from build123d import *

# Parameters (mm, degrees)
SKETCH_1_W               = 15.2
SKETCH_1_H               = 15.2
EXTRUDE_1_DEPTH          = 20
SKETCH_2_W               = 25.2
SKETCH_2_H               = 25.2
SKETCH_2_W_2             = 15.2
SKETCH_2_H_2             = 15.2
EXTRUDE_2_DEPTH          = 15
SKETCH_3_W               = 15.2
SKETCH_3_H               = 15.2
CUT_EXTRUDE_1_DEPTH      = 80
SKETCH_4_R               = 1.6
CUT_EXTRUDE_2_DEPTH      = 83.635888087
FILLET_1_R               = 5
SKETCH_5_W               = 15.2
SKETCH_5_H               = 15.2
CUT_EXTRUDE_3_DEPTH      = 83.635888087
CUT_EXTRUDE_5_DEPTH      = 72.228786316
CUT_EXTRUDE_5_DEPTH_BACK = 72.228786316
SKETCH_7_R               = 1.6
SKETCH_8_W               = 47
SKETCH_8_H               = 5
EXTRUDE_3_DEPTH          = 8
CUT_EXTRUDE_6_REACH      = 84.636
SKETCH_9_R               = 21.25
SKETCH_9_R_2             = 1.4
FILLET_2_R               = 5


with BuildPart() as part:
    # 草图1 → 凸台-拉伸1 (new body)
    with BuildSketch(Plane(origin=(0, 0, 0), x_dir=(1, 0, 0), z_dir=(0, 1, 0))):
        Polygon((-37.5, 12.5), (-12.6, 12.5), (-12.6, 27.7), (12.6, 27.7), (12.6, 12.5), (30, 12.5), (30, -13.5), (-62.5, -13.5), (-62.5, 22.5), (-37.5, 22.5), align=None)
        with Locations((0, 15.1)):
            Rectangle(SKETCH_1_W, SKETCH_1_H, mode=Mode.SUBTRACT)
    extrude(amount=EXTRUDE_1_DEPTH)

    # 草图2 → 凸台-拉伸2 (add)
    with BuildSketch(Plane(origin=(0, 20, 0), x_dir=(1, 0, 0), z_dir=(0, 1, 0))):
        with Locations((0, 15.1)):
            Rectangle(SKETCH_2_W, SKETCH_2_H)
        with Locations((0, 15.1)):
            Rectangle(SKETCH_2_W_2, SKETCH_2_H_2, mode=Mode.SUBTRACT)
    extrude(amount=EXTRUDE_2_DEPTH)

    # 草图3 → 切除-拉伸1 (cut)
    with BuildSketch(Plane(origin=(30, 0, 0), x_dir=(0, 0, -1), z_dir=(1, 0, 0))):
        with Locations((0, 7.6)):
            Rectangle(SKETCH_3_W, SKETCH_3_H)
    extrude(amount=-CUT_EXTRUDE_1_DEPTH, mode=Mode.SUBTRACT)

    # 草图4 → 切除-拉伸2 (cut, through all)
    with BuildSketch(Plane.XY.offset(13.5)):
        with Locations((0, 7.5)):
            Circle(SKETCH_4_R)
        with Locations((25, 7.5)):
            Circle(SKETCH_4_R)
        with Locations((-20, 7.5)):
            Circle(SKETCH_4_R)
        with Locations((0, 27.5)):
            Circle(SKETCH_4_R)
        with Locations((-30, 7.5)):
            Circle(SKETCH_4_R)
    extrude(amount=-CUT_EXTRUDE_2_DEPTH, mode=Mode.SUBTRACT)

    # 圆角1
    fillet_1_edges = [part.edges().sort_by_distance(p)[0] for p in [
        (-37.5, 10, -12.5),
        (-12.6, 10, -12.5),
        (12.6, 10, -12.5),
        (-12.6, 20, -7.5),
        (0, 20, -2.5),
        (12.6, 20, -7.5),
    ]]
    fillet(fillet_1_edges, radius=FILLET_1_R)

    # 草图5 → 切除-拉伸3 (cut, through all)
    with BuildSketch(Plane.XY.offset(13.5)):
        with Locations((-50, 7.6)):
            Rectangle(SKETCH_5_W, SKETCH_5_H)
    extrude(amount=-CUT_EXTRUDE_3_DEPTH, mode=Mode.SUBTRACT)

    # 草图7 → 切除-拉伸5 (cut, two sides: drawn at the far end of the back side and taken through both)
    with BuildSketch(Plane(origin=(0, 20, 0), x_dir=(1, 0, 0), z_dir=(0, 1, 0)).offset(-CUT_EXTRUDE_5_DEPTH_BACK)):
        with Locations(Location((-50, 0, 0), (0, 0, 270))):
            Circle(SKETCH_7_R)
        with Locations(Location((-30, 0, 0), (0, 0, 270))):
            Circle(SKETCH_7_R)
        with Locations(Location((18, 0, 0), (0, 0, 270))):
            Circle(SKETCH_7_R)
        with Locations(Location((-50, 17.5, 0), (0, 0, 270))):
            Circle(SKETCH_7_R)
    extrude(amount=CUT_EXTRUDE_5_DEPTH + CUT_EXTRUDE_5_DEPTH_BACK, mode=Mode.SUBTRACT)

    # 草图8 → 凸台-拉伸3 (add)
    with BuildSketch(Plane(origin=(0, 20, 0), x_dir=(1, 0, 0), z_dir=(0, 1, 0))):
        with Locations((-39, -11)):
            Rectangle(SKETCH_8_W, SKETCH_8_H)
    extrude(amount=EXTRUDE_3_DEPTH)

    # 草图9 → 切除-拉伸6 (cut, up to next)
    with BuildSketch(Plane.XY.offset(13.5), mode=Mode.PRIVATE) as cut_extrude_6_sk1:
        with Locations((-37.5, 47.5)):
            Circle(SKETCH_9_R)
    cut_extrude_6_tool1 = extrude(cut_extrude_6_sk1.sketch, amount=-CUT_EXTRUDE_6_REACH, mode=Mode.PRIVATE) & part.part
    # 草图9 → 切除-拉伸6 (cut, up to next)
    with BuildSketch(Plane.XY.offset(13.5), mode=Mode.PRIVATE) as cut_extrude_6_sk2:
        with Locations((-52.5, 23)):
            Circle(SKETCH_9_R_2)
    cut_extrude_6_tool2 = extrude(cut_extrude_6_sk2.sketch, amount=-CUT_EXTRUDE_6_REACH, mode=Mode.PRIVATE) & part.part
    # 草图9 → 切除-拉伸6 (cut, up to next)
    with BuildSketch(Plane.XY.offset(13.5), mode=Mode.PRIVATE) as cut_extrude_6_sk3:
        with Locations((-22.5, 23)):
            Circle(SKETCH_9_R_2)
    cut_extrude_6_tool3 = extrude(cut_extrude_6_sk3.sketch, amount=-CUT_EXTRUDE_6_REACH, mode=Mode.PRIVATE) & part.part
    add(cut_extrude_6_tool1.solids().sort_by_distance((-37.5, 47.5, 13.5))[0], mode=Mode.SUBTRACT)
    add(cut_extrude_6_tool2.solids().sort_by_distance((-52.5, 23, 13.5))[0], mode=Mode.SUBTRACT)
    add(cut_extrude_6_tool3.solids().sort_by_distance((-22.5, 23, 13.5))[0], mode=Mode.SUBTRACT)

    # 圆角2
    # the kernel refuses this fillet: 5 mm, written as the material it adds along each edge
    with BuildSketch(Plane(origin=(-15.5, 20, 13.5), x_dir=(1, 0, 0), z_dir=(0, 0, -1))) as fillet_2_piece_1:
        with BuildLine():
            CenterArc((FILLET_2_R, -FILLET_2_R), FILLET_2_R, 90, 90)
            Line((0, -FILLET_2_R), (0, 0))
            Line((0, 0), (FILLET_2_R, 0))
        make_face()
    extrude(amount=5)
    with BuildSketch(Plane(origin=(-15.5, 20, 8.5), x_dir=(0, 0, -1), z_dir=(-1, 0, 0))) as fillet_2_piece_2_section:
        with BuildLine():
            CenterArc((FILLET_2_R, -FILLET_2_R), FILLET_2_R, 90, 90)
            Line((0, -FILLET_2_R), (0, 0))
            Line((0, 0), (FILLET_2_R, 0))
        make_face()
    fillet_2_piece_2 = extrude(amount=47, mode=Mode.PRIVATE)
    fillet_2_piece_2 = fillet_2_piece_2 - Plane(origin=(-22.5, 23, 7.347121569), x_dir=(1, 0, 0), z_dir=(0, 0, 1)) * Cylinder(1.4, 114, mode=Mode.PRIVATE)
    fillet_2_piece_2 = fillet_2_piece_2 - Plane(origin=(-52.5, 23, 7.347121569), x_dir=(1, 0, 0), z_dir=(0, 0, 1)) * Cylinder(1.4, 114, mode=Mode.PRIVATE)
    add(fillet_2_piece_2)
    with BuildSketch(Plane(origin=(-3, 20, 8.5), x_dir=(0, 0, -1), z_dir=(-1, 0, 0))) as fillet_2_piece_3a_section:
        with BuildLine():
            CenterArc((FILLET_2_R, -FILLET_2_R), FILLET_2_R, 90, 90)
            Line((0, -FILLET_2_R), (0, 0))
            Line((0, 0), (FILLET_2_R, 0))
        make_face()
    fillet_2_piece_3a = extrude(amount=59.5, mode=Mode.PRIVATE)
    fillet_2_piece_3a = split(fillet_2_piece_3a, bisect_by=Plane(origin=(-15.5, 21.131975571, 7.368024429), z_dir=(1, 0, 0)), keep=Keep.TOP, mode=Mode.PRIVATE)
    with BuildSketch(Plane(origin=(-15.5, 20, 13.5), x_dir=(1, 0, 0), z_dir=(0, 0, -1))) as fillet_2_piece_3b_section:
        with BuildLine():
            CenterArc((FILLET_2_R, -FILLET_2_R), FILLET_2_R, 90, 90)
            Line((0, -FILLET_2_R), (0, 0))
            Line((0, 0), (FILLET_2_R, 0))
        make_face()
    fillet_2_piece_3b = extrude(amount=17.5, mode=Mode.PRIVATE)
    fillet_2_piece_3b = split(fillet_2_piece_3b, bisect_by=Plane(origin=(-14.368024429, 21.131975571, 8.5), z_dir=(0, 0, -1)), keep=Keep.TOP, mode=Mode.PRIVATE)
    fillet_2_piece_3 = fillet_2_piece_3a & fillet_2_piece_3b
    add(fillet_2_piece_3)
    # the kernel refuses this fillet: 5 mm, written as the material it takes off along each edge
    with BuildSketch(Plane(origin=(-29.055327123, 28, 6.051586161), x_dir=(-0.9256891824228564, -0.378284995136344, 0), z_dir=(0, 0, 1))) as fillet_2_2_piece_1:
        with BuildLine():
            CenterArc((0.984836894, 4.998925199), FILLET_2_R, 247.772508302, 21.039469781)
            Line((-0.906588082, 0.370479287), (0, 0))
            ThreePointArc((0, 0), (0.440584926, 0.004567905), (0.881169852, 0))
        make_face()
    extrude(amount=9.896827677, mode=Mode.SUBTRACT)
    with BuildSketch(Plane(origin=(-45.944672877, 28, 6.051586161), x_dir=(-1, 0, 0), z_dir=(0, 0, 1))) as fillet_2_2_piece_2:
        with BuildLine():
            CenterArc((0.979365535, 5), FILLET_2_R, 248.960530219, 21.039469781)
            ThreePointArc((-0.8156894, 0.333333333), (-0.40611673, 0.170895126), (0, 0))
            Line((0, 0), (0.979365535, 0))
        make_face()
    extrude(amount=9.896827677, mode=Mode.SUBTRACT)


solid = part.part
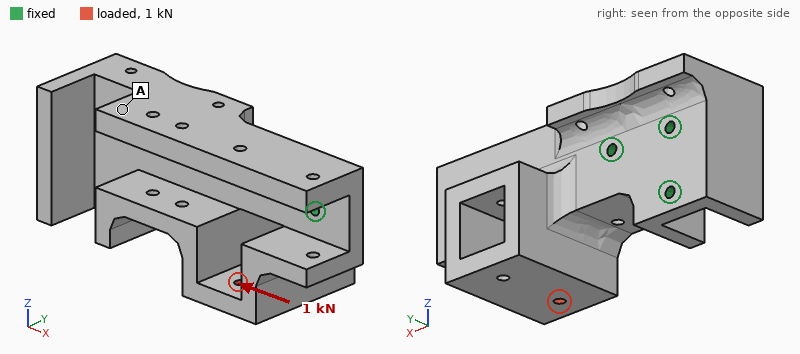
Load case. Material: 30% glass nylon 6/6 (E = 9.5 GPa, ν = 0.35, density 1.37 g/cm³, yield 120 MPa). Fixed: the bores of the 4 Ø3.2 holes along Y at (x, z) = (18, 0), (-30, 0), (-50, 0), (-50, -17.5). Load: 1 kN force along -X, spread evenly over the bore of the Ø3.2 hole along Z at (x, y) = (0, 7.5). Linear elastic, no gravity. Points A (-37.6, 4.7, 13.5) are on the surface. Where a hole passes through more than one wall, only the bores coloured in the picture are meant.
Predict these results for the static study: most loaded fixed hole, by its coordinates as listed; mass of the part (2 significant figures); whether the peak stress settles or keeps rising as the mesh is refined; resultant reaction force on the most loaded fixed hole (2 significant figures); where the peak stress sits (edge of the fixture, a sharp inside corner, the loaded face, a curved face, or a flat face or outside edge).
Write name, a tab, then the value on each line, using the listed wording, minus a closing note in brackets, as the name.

most loaded fixed hole, by its coordinates as listed	(18, 0)
mass of the part	54 g
whether the peak stress settles or keeps rising as the mesh is refined	keeps rising
resultant reaction force on the most loaded fixed hole	730 N
where the peak stress sits	a sharp inside corner
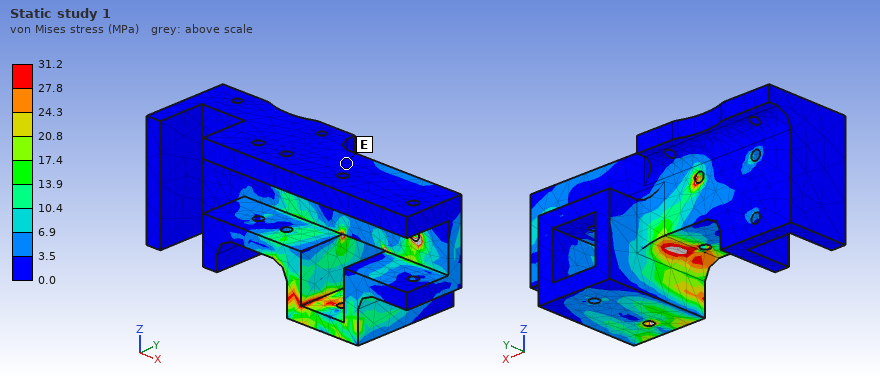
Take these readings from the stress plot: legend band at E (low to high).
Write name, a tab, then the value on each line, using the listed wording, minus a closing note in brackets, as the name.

legend band at E	0.0 to 3.5 MPa
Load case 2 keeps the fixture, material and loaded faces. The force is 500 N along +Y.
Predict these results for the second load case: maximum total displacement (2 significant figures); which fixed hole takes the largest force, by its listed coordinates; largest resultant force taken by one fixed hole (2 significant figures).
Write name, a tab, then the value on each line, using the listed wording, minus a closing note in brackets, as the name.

maximum total displacement	0.64 mm
which fixed hole takes the largest force, by its listed coordinates	(18, 0)
largest resultant force taken by one fixed hole	340 N
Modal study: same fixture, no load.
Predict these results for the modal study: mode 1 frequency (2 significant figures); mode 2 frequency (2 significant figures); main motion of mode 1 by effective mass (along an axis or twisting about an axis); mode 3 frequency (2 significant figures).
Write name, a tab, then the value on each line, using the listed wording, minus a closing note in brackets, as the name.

mode 1 frequency	1400 Hz
mode 2 frequency	3100 Hz
main motion of mode 1 by effective mass	along Y
mode 3 frequency	3900 Hz
